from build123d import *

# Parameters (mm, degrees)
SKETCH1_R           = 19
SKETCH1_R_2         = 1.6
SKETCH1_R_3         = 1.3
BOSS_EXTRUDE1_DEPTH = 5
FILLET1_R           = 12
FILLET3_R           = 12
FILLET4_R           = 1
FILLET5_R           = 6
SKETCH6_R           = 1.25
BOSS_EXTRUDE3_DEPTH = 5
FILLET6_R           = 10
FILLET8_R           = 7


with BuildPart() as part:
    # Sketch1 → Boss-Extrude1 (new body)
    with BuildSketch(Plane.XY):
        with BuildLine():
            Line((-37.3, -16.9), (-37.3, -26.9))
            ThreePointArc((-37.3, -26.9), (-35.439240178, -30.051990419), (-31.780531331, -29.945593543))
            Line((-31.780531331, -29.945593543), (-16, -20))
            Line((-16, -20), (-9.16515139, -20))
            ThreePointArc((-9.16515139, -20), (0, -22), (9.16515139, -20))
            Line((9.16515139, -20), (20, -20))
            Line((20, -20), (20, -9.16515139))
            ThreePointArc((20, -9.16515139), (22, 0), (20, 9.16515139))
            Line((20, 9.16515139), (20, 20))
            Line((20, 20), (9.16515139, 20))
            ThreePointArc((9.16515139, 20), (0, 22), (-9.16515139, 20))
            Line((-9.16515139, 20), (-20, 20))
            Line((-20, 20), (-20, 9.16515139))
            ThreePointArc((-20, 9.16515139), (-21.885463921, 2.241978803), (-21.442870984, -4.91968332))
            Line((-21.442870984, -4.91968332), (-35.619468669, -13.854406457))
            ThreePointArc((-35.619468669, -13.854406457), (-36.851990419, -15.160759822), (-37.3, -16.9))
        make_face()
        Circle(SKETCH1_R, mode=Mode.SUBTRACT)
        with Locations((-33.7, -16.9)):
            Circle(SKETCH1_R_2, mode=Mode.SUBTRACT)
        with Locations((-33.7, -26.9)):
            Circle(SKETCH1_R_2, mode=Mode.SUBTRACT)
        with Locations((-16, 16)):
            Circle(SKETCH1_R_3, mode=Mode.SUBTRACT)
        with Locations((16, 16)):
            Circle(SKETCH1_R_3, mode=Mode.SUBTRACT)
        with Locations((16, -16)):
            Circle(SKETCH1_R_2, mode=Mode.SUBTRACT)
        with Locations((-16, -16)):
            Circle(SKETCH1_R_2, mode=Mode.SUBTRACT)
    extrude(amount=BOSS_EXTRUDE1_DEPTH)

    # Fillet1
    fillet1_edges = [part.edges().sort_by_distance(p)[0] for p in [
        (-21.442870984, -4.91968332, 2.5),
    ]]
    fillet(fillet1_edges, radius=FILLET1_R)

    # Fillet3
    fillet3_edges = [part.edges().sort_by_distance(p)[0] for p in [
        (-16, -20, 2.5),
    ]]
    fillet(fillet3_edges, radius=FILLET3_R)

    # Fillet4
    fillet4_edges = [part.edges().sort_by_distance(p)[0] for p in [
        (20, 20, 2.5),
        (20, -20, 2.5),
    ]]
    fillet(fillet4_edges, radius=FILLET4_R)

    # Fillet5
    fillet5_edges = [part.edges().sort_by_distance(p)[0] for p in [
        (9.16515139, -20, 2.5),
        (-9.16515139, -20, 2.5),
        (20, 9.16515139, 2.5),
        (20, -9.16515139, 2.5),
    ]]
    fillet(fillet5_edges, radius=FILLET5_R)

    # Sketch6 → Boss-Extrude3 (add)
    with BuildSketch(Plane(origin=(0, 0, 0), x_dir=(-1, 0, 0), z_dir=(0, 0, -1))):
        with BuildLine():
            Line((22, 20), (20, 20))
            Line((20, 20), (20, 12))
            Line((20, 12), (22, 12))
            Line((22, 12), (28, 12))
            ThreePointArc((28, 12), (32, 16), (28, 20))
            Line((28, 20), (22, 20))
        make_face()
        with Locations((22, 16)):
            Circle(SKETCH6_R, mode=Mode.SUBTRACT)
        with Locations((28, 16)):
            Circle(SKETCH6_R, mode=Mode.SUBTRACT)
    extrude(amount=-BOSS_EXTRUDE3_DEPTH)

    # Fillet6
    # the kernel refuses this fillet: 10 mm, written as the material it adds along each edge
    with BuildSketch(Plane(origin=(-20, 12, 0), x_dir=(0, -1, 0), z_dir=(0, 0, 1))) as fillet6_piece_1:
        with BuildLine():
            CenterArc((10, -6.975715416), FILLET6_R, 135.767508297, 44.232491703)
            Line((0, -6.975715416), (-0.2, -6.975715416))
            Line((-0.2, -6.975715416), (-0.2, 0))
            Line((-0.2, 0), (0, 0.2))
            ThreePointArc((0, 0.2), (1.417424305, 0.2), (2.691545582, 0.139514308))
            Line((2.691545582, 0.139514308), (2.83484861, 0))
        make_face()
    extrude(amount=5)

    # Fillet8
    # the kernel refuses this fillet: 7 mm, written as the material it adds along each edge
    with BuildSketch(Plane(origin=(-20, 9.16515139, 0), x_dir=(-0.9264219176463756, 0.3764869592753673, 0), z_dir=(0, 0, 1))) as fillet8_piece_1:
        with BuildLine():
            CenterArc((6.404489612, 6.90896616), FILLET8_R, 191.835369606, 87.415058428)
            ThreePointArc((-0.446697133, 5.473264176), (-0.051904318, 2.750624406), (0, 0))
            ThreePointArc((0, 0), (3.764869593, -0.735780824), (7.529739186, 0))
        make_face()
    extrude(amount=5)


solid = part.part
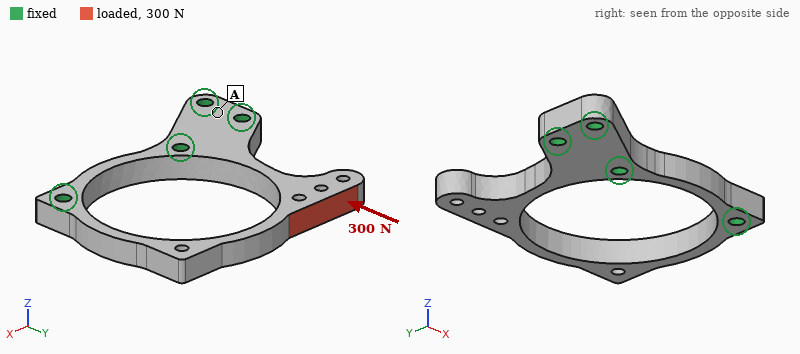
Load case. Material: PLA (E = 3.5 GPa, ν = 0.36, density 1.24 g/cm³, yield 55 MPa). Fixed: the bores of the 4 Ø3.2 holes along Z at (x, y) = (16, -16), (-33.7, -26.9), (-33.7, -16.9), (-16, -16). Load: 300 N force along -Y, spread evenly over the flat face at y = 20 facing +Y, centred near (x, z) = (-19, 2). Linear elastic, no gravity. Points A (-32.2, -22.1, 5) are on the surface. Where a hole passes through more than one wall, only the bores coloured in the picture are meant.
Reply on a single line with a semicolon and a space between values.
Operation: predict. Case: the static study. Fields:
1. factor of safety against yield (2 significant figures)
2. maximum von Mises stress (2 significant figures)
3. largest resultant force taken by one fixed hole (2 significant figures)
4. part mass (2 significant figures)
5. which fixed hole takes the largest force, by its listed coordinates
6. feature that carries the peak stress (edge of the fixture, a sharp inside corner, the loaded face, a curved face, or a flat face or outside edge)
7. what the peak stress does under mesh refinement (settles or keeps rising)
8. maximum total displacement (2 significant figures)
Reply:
1.8; 30 MPa; 200 N; 5.8 g; (-16, -16); a curved face; settles; 0.36 mm
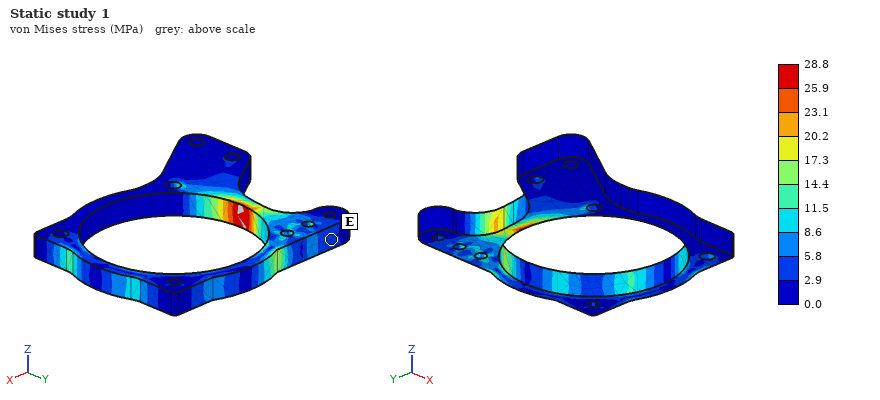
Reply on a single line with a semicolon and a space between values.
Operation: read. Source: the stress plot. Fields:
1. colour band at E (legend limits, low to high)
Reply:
2.9 to 5.8 MPa
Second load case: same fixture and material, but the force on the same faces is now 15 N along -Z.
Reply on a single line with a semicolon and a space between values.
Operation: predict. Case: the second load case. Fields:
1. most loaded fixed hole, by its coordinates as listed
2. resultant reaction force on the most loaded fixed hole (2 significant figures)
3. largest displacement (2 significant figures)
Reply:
(-16, -16); 14 N; 0.91 mm
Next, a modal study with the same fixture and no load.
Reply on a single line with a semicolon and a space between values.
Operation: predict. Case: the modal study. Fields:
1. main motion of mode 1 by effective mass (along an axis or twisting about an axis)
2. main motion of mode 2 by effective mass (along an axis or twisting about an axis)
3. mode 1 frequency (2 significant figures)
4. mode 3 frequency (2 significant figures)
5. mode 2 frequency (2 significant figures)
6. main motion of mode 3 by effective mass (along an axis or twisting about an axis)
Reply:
along Z; twisting about Y; 620 Hz; 1100 Hz; 1000 Hz; along X
